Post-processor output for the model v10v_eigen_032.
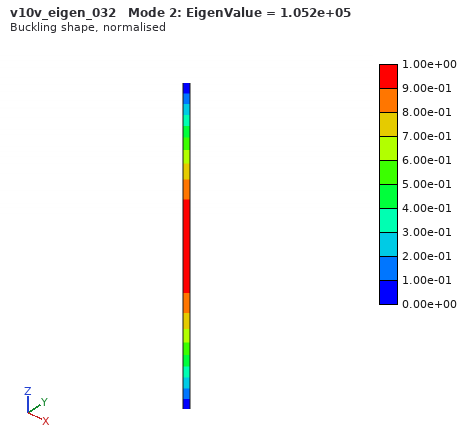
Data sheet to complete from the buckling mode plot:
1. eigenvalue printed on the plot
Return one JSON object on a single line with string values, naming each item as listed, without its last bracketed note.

{"eigenvalue printed on the plot": "1.052e+05"}
